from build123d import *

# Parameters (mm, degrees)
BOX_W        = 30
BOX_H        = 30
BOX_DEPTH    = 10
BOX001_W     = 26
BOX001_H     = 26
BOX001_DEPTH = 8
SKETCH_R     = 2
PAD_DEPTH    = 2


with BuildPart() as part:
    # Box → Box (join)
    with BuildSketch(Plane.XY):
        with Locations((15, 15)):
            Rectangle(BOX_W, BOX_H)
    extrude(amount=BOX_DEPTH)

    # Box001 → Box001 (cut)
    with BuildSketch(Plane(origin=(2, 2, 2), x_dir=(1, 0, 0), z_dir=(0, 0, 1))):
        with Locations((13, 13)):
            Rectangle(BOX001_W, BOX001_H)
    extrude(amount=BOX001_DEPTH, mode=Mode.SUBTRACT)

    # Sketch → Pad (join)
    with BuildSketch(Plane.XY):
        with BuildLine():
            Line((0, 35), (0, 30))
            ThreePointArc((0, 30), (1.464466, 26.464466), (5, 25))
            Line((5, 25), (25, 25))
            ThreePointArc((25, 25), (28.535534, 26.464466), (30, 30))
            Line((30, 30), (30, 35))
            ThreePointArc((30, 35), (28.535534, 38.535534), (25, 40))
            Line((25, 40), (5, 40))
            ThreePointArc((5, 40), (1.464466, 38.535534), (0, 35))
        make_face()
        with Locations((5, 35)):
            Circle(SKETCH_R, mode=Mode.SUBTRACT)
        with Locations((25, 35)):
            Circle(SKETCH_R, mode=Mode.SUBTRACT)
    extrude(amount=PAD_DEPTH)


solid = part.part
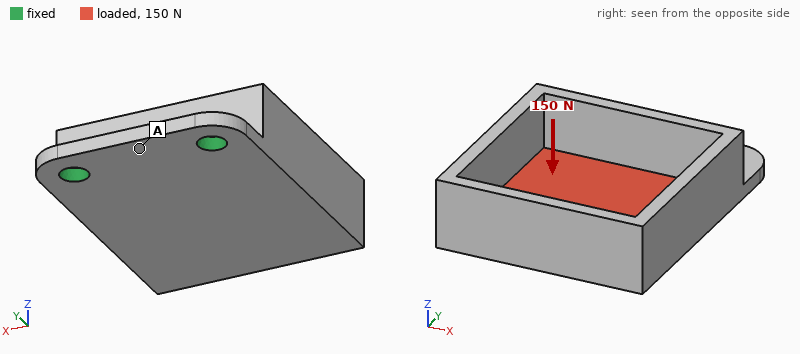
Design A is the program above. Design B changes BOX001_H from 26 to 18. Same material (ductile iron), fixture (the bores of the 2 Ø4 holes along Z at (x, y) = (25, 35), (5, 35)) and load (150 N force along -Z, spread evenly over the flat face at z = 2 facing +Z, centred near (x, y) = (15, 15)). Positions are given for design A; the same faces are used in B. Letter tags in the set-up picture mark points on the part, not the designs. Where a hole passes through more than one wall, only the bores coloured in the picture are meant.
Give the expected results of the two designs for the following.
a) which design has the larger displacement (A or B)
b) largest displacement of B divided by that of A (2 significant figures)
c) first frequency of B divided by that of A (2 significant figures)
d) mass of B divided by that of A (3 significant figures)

A
0.90
0.86
1.40
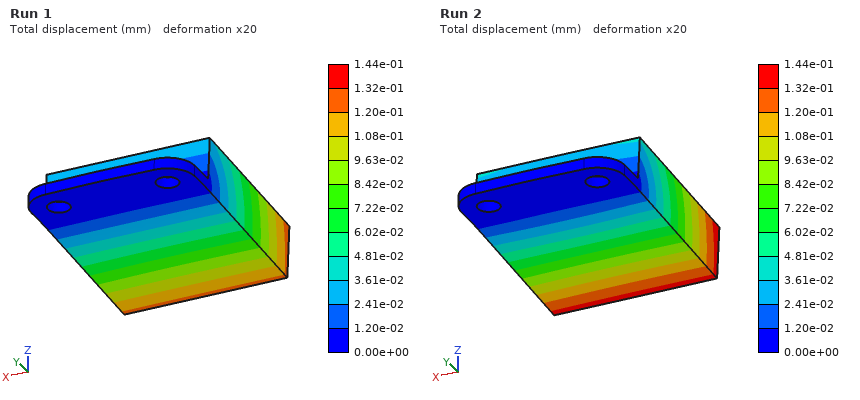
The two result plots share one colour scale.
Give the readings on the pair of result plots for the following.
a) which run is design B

Run 1
